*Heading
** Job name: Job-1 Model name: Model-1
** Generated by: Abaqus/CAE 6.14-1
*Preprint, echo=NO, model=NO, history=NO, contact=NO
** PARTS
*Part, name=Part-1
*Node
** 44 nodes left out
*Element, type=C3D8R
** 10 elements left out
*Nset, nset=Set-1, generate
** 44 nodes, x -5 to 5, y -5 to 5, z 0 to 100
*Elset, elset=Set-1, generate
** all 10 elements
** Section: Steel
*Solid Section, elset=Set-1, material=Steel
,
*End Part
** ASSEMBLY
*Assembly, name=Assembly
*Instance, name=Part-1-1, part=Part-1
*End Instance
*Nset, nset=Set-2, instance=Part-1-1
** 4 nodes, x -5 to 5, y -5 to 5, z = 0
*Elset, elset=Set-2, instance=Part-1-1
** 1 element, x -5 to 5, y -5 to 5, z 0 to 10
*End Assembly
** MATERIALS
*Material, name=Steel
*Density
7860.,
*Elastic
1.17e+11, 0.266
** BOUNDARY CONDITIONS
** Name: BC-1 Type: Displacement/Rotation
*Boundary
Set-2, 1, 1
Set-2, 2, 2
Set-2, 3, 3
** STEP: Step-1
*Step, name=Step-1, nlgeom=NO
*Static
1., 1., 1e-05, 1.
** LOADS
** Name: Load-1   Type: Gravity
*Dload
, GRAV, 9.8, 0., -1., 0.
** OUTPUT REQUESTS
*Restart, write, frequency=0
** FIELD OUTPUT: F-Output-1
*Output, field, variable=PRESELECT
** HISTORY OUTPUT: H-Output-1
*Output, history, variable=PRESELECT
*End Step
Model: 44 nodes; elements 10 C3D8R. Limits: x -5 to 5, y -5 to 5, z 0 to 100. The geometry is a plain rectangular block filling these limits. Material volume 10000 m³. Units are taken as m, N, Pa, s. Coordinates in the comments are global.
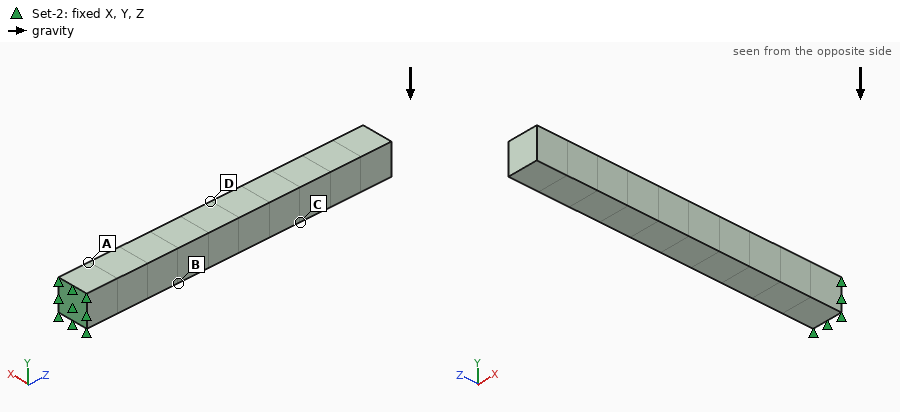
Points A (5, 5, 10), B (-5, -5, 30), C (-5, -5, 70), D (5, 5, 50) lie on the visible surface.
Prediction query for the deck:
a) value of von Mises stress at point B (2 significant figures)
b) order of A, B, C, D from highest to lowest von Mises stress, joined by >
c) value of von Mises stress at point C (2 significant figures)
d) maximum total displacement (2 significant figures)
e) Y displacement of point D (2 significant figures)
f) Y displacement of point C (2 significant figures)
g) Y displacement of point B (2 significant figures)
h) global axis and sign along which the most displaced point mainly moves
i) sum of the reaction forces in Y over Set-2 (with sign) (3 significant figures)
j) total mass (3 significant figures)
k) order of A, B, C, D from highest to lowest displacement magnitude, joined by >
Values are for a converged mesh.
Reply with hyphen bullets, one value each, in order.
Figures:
- 1.1e+08 Pa
- A > B > D > C
- 2.1e+07 Pa
- 0.99 m
- -0.35 m
- -0.60 m
- -0.15 m
- -Y
- 7.70e+08 N
- 7.86e+07 kg
- C > D > B > A
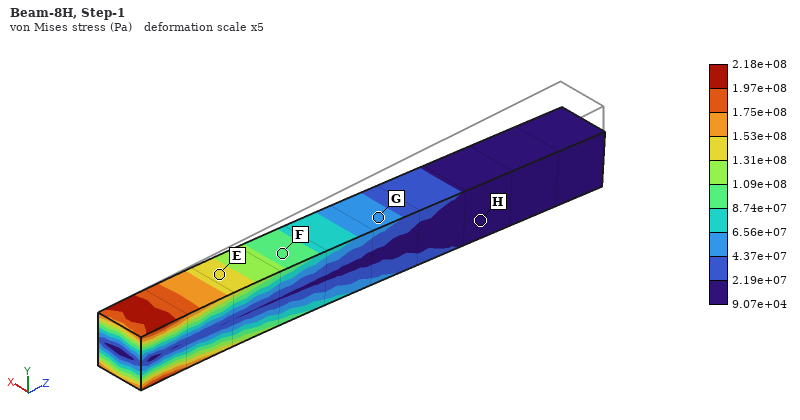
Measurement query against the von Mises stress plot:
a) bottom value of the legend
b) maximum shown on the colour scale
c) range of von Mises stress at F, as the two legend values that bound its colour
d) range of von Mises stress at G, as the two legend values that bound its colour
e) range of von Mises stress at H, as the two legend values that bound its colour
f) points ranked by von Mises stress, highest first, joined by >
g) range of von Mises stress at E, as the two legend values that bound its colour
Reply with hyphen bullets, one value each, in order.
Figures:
- 9.07e+04 Pa
- 2.18e+08 Pa
- 8.74e+07 to 1.09e+08 Pa
- 4.37e+07 to 6.56e+07 Pa
- 9.07e+04 to 2.19e+07 Pa
- E > F > G > H
- 1.31e+08 to 1.53e+08 Pa
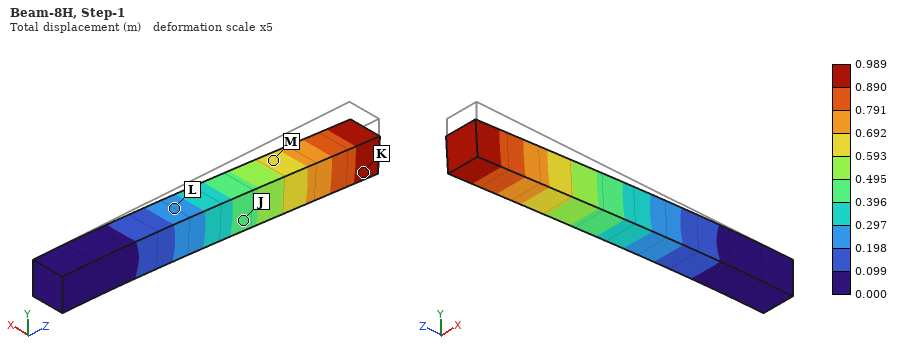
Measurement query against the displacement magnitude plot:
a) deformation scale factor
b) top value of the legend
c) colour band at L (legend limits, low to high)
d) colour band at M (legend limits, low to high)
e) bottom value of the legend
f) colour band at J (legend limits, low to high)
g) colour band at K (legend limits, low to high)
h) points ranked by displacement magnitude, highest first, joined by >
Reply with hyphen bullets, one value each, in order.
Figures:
- 5
- 0.989 m
- 0.198 to 0.297 m
- 0.593 to 0.692 m
- 0.000 m
- 0.396 to 0.495 m
- 0.890 to 0.989 m
- K > M > J > L
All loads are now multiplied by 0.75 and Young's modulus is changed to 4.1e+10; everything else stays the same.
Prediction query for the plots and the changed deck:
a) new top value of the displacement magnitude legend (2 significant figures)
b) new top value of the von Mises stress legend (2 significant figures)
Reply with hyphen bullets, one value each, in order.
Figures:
- 2.1 m
- 1.6e+08 Pa
